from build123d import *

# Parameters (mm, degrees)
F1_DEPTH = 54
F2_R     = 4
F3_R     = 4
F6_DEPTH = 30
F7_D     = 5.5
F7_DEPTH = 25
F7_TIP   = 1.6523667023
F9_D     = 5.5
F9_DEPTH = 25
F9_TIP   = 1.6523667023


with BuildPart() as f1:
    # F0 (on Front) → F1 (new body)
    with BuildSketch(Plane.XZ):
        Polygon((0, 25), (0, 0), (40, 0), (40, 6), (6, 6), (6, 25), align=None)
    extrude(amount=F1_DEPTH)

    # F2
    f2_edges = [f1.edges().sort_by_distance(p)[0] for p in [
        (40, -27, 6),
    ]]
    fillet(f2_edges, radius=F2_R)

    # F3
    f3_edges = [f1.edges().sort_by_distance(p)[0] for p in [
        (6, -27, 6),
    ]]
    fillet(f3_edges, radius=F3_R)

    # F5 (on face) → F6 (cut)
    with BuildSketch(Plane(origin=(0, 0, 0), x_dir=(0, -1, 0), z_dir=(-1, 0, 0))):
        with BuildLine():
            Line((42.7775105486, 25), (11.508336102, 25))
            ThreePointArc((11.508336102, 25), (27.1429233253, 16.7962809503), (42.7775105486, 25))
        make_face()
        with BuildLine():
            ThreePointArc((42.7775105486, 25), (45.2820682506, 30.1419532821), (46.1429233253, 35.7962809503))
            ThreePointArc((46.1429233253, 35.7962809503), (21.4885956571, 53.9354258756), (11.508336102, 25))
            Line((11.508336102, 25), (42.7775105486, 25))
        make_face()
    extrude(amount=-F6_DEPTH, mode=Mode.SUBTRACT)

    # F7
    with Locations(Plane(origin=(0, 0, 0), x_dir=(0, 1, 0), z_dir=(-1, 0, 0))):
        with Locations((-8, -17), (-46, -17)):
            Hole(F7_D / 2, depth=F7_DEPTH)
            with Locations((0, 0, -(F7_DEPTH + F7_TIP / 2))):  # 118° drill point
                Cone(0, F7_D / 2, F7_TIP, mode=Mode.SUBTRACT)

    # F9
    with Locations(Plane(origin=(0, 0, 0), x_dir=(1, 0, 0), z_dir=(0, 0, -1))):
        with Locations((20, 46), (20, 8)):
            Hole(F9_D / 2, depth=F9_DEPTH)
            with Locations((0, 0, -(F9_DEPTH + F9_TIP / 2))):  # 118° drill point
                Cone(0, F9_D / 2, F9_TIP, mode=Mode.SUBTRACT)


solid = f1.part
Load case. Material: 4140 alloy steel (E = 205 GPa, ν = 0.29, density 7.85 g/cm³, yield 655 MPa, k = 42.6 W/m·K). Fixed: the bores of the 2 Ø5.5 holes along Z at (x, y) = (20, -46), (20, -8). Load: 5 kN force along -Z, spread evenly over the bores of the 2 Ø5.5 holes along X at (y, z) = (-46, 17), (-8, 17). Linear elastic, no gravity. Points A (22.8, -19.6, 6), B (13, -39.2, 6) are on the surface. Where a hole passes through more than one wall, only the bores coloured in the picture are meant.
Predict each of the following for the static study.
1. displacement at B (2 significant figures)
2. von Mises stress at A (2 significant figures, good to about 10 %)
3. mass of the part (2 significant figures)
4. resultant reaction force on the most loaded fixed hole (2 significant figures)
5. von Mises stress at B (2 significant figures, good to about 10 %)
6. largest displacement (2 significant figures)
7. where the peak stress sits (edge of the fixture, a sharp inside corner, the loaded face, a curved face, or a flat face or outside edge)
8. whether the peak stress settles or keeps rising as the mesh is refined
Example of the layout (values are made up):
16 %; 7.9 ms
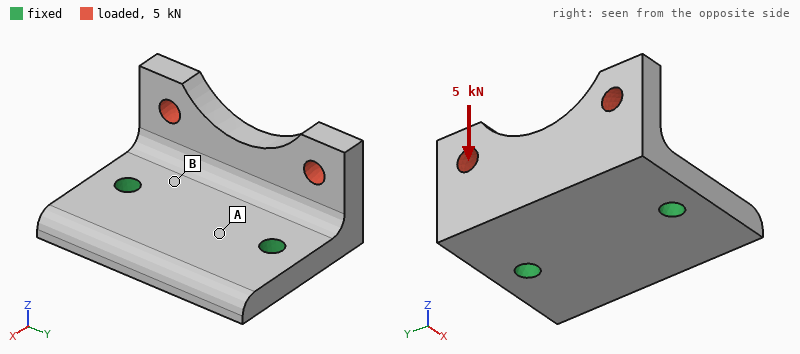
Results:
0.016 mm; 58 MPa; 140 g; 2.5 kN; 130 MPa; 0.10 mm; edge of the fixture; keeps rising
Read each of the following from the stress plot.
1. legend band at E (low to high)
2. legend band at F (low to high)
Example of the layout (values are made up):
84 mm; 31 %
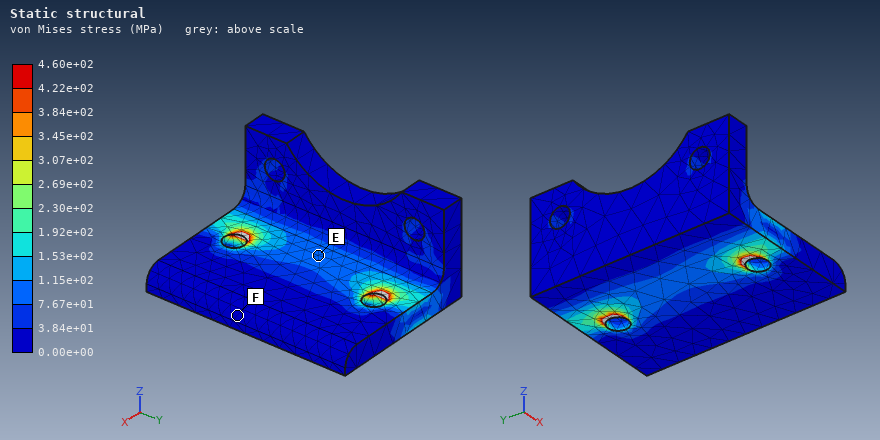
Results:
7.67e+01 to 1.15e+02 MPa; 0.00e+00 to 3.84e+01 MPa
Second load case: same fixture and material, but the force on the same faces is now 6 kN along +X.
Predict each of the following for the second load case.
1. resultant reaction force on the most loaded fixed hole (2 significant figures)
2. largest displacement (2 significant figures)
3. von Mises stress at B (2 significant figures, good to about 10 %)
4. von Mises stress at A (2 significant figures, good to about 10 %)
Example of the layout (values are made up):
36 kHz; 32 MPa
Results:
3.0 kN; 0.20 mm; 240 MPa; 77 MPa
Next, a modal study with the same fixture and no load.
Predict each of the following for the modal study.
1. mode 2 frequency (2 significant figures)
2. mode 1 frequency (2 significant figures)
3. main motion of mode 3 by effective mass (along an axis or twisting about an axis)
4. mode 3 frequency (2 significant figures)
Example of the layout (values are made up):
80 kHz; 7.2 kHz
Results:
8000 Hz; 5000 Hz; along Z; 11 kHz
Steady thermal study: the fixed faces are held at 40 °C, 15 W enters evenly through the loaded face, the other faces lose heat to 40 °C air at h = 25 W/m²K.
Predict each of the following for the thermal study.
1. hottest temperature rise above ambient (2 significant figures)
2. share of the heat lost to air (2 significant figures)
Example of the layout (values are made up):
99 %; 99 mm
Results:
37 K; 15 %
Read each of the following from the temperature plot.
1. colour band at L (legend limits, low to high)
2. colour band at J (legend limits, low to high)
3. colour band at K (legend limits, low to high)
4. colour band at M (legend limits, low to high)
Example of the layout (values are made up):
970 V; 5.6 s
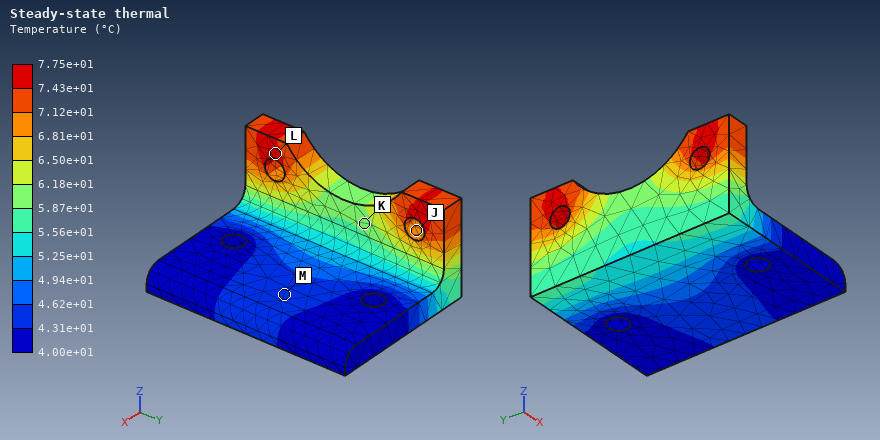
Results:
7.43e+01 to 7.75e+01 °C; 6.81e+01 to 7.12e+01 °C; 5.87e+01 to 6.18e+01 °C; 4.31e+01 to 4.62e+01 °C
